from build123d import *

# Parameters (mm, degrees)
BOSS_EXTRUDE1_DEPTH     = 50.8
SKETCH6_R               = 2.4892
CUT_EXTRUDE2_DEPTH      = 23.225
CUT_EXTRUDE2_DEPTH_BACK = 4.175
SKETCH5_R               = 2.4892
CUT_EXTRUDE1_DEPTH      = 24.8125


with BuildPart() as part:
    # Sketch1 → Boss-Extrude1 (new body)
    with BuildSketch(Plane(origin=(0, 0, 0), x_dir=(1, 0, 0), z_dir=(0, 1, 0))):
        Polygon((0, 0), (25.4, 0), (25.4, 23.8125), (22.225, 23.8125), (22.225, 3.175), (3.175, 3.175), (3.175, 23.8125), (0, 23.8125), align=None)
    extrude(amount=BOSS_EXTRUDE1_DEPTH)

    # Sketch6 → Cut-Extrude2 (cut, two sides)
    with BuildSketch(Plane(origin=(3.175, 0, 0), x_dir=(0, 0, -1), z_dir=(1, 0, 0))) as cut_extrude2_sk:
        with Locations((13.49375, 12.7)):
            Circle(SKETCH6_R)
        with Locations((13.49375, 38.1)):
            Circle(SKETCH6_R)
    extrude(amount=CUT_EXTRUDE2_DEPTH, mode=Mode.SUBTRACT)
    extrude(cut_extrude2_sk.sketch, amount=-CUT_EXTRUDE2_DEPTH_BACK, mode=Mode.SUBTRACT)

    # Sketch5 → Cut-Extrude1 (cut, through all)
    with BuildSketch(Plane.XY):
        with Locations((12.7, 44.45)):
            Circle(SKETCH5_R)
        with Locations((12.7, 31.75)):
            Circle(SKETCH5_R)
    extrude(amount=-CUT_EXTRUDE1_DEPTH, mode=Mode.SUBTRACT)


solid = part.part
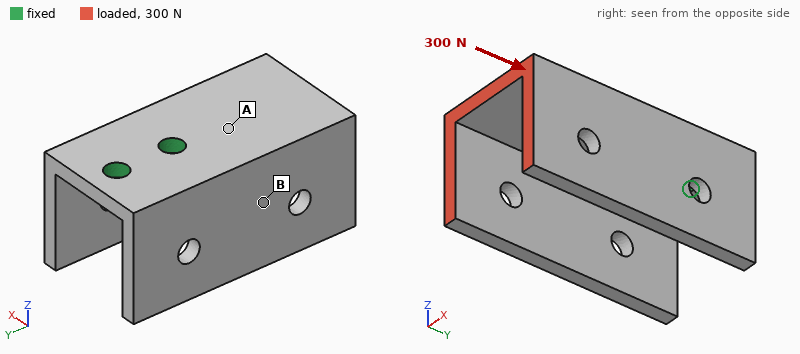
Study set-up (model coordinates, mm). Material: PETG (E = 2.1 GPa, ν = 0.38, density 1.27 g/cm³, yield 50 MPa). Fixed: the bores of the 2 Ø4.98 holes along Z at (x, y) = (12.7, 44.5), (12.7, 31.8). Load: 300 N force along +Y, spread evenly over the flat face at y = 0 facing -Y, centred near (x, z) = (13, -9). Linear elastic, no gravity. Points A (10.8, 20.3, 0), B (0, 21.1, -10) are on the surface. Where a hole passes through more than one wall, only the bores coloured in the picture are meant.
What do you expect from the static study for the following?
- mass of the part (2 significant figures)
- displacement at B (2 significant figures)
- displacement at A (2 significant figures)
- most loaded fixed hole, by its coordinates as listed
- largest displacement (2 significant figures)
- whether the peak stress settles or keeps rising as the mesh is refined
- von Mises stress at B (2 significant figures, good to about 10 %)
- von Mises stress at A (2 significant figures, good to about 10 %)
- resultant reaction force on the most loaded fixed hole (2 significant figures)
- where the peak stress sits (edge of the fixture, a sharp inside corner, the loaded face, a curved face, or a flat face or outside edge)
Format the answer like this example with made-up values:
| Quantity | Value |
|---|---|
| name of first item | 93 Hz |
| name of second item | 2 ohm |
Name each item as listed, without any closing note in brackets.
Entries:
| Quantity | Value |
|---|---|
| mass of the part | 13 g |
| displacement at B | 0.24 mm |
| displacement at A | 0.15 mm |
| most loaded fixed hole, by its coordinates as listed | (12.7, 31.8) |
| largest displacement | 0.61 mm |
| whether the peak stress settles or keeps rising as the mesh is refined | keeps rising |
| von Mises stress at B | 2.1 MPa |
| von Mises stress at A | 5.6 MPa |
| resultant reaction force on the most loaded fixed hole | 230 N |
| where the peak stress sits | edge of the fixture |
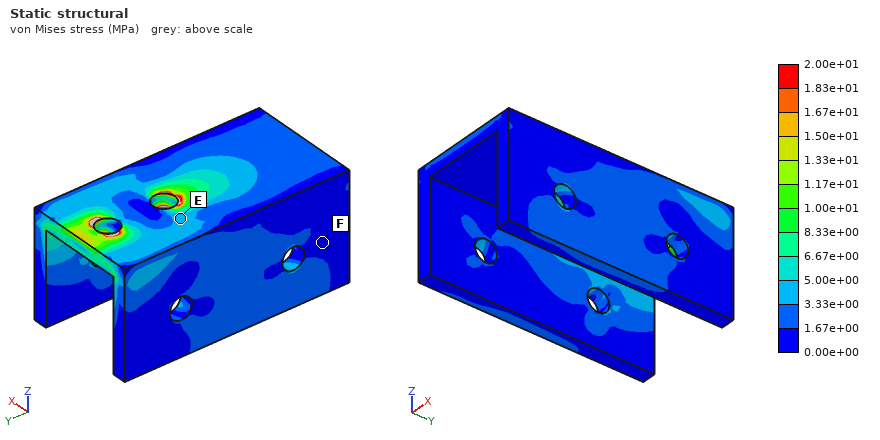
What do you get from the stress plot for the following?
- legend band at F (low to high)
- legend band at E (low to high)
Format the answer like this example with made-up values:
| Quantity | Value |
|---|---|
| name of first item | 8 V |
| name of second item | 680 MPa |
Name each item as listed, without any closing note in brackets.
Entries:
| Quantity | Value |
|---|---|
| legend band at F | 0.00e+00 to 1.67e+00 MPa |
| legend band at E | 3.33e+00 to 5.00e+00 MPa |
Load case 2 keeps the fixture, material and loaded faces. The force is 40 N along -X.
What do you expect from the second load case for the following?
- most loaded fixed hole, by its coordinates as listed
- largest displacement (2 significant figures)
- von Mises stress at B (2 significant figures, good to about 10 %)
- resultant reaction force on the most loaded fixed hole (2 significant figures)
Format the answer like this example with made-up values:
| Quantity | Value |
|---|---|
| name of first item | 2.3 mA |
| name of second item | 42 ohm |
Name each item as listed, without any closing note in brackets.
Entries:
| Quantity | Value |
|---|---|
| most loaded fixed hole, by its coordinates as listed | (12.7, 31.8) |
| largest displacement | 0.64 mm |
| von Mises stress at B | 2.0 MPa |
| resultant reaction force on the most loaded fixed hole | 100 N |
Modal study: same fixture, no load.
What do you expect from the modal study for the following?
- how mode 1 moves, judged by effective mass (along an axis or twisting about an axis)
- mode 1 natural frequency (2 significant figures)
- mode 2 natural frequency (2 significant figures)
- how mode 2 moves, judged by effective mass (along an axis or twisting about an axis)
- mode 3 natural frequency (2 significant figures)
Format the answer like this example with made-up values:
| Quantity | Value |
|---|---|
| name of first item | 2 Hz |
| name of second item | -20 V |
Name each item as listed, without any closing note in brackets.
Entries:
| Quantity | Value |
|---|---|
| how mode 1 moves, judged by effective mass | along X |
| mode 1 natural frequency | 590 Hz |
| mode 2 natural frequency | 780 Hz |
| how mode 2 moves, judged by effective mass | along Z |
| mode 3 natural frequency | 900 Hz |
